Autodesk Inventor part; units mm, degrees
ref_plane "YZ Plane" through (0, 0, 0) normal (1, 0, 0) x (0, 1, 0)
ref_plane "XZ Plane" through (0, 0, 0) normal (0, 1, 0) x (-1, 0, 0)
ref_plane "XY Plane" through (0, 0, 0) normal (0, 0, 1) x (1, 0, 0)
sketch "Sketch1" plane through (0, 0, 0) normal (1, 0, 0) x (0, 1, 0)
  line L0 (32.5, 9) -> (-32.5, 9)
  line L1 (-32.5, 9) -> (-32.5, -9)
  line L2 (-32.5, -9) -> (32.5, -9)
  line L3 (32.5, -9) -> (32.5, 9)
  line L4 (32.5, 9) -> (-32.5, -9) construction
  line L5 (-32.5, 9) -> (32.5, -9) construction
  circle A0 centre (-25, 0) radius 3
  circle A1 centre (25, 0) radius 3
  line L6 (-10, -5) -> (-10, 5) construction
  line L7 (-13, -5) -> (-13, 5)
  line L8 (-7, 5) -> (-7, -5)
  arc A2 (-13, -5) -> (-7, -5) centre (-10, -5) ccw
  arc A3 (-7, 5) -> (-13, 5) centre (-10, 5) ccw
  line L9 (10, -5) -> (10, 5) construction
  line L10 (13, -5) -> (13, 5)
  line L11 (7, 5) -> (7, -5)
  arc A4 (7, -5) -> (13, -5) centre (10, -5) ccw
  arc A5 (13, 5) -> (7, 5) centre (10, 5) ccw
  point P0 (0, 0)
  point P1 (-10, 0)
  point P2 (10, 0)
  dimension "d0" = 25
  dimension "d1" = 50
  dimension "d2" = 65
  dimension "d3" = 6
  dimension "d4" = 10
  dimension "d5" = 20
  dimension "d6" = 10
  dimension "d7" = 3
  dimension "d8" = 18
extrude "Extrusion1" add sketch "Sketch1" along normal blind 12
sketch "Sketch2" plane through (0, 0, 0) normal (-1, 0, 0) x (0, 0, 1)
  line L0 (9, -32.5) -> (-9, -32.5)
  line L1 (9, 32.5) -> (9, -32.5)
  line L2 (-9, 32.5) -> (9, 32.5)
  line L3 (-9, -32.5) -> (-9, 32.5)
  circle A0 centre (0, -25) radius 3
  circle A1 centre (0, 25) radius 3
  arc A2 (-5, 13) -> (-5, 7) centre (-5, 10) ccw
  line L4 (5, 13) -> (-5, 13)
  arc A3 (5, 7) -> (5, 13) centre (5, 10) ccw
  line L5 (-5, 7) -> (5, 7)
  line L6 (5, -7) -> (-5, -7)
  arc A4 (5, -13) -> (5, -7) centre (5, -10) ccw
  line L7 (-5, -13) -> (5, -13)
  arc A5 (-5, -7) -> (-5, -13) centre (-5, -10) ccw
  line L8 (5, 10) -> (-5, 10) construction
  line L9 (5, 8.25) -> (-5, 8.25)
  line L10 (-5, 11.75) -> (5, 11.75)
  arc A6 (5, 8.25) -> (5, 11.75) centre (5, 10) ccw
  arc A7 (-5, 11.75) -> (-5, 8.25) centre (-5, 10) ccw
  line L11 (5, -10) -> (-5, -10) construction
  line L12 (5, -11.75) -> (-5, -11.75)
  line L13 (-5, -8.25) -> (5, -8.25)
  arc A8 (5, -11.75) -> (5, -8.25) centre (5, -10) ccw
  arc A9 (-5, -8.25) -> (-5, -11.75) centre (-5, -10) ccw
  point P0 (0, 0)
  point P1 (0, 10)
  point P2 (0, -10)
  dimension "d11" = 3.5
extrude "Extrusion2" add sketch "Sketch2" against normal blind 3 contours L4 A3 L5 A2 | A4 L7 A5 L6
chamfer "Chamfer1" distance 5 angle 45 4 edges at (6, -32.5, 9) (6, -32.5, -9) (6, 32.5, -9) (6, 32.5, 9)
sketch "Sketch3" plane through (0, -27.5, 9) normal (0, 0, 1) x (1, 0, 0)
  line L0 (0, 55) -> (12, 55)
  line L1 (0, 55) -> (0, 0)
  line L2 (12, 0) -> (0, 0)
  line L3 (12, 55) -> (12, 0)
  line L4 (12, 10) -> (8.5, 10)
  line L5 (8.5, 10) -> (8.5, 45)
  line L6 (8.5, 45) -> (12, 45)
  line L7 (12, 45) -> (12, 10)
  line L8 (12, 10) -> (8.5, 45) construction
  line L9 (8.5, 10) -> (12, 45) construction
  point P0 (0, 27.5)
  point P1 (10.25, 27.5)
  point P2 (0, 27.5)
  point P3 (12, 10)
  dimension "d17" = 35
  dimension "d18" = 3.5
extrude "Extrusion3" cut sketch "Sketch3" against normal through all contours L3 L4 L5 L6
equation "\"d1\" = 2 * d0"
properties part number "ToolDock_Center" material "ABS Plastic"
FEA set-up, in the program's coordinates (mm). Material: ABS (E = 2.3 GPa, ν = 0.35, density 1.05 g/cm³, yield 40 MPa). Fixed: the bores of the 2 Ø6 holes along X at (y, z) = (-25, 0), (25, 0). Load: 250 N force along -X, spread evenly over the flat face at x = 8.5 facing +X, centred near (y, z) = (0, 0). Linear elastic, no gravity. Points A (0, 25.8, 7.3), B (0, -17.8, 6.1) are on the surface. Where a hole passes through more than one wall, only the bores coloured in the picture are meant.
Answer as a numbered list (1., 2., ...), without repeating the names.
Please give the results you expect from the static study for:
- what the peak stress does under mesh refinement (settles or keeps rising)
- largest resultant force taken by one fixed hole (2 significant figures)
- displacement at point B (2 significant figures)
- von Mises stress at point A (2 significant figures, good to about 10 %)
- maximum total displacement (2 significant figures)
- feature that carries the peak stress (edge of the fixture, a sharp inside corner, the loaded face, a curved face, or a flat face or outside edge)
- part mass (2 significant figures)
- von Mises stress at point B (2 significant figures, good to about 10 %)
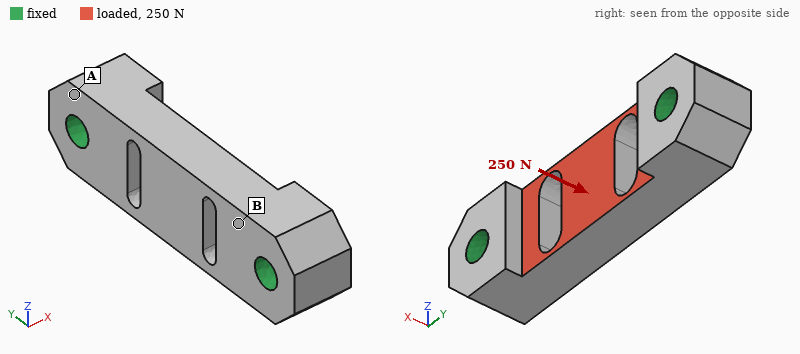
1. keeps rising
2. 130 N
3. 15 µm
4. 1.1 MPa
5. 86 µm
6. a sharp inside corner
7. 9.8 g
8. 2.9 MPa
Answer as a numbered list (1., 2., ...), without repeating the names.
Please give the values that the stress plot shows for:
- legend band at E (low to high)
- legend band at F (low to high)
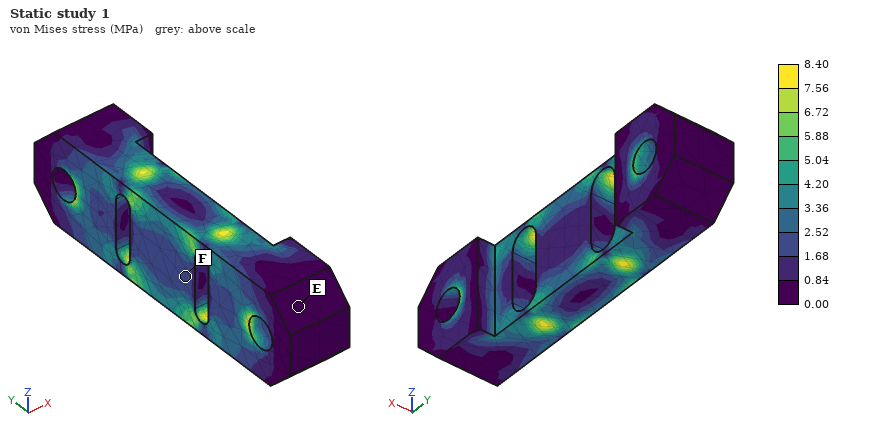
1. 0.00 to 0.84 MPa
2. 1.68 to 2.52 MPa
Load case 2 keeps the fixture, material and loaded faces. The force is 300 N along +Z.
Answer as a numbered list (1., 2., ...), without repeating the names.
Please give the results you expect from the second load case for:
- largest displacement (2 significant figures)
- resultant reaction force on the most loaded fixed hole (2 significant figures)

1. 0.19 mm
2. 150 N
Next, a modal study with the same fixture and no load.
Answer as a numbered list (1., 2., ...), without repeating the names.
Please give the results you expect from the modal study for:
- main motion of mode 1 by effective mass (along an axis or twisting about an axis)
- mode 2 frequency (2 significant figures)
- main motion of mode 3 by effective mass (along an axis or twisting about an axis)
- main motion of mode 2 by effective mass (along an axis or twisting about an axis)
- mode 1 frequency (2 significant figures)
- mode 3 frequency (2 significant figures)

1. along Z
2. 4400 Hz
3. twisting about Y
4. along X
5. 3900 Hz
6. 6700 Hz
